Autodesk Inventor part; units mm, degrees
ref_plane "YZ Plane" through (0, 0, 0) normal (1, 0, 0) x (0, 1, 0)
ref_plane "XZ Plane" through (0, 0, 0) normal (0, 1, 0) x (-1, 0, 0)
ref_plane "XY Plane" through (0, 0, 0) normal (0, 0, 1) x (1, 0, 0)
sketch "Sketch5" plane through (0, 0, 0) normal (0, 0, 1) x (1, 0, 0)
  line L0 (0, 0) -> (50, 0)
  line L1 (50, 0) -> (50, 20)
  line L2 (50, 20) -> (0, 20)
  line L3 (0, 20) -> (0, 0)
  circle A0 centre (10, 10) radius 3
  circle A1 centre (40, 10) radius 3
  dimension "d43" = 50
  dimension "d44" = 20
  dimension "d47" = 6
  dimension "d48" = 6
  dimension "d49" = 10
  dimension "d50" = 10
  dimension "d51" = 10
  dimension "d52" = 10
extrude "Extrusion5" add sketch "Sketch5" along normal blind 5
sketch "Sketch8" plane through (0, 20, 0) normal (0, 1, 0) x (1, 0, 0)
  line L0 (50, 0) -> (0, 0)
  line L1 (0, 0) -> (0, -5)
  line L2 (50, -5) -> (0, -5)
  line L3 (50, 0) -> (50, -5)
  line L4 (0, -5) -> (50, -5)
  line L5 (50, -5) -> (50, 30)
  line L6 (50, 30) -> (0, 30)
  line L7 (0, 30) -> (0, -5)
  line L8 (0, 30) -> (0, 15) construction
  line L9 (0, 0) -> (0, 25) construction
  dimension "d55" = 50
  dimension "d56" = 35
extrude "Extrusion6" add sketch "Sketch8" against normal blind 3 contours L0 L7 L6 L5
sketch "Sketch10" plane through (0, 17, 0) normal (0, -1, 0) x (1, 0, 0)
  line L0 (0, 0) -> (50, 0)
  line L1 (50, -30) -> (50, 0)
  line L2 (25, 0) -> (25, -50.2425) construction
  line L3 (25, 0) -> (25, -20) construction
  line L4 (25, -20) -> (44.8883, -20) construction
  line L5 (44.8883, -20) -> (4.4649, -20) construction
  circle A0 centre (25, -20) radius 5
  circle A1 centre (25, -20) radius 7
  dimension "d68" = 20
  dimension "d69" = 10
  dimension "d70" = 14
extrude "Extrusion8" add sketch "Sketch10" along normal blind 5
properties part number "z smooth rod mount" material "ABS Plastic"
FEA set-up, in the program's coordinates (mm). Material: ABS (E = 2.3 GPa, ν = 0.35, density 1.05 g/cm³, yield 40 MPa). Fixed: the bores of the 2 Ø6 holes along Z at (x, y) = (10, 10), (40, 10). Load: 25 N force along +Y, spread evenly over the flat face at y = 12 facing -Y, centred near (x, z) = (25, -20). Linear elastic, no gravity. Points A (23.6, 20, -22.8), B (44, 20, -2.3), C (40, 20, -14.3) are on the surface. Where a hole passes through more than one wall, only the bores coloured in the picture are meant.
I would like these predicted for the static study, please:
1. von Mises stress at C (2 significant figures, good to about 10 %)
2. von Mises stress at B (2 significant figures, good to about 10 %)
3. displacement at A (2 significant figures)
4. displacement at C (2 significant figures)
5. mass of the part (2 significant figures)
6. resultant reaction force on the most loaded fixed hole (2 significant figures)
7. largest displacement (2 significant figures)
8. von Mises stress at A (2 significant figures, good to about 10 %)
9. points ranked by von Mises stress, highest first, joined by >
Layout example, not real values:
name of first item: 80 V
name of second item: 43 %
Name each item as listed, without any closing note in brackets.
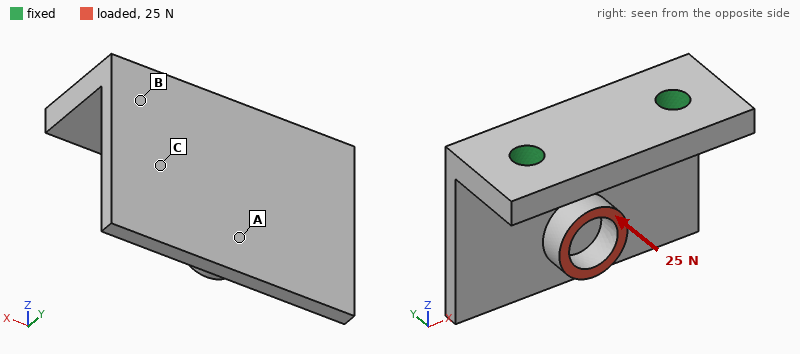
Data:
von Mises stress at C: 2.2 MPa
von Mises stress at B: 4.8 MPa
displacement at A: 0.47 mm
displacement at C: 0.23 mm
mass of the part: 10 g
resultant reaction force on the most loaded fixed hole: 13 N
largest displacement: 0.65 mm
von Mises stress at A: 1.1 MPa
points ranked by von Mises stress, highest first, joined by >: B > C > A
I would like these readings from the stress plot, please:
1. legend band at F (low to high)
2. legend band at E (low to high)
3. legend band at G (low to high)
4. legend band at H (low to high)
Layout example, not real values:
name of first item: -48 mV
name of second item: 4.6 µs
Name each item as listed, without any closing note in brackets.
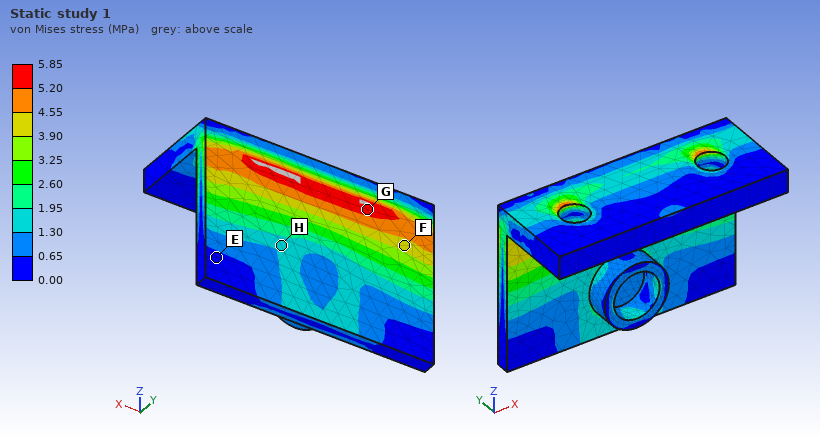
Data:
legend band at F: 3.90 to 4.55 MPa
legend band at E: 0.00 to 0.65 MPa
legend band at G: 5.20 to 5.85 MPa
legend band at H: 1.30 to 1.95 MPa
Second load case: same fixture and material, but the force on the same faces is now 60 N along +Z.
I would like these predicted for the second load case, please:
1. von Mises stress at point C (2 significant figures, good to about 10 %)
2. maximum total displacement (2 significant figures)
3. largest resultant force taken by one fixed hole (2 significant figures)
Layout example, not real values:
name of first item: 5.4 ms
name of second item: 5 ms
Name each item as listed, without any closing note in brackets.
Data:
von Mises stress at point C: 3.5 MPa
maximum total displacement: 0.66 mm
largest resultant force taken by one fixed hole: 31 N
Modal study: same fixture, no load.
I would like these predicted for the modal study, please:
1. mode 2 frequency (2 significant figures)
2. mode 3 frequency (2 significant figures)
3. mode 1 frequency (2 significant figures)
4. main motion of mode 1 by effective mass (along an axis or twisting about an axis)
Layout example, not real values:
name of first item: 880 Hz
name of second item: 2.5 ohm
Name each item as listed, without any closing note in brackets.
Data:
mode 2 frequency: 1300 Hz
mode 3 frequency: 2800 Hz
mode 1 frequency: 650 Hz
main motion of mode 1 by effective mass: along Y
